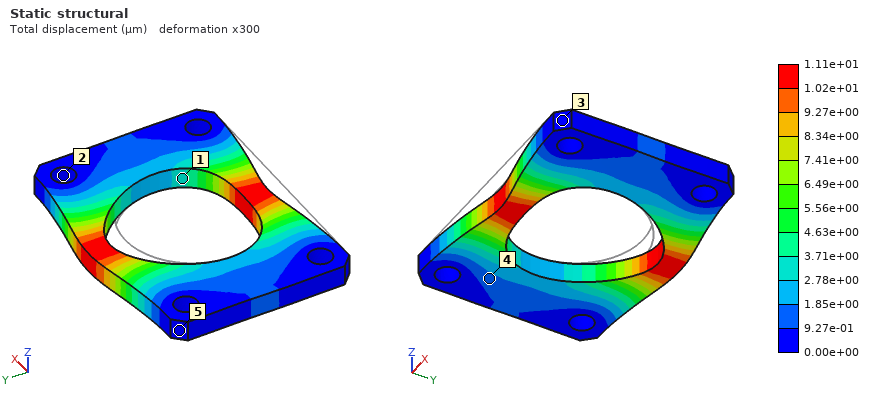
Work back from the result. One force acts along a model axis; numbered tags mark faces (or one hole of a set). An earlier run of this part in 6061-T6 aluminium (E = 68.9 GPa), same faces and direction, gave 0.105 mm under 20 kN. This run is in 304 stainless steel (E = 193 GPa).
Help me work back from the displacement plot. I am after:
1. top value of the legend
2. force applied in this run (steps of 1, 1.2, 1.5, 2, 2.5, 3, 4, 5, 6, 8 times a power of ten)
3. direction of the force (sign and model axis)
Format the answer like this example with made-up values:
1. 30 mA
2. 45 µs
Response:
1. 1.11e+01 µm
2. 6 kN
3. +Y
